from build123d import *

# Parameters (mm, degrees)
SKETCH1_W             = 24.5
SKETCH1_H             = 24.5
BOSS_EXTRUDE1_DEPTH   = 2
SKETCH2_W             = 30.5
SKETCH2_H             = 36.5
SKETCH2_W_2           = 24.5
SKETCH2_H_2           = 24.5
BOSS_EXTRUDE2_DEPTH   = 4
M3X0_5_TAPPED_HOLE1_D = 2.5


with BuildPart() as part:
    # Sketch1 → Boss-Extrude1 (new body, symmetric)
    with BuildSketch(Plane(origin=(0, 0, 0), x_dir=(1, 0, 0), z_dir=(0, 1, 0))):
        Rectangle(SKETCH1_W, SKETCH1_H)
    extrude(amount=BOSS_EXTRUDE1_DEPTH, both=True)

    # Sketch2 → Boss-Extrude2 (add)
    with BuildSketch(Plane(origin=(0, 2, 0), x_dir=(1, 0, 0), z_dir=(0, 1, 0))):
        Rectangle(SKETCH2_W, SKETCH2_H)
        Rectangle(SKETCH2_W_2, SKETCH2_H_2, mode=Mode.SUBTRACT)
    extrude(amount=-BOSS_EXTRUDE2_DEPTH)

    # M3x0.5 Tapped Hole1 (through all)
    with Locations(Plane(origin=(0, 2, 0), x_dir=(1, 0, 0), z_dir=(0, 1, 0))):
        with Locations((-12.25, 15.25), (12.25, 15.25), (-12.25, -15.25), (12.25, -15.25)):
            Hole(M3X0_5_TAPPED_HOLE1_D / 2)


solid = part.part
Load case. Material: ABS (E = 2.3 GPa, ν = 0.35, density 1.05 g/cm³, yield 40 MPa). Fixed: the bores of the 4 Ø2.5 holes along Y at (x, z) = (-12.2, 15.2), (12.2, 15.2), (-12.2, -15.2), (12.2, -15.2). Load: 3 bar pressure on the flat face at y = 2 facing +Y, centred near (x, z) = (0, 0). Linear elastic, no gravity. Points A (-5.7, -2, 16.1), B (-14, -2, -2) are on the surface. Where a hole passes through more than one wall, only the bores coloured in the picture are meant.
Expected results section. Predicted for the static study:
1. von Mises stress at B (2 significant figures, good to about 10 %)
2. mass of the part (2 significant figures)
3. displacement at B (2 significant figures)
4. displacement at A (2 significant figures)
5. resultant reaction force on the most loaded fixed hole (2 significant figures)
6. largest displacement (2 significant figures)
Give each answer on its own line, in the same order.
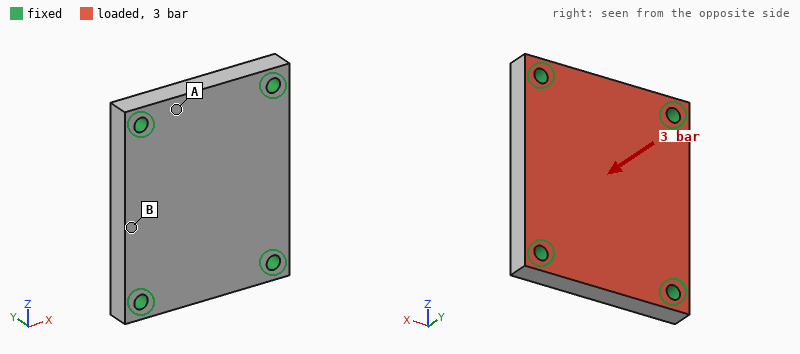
5.3 MPa
4.6 g
0.081 mm
0.027 mm
82 N
0.11 mm
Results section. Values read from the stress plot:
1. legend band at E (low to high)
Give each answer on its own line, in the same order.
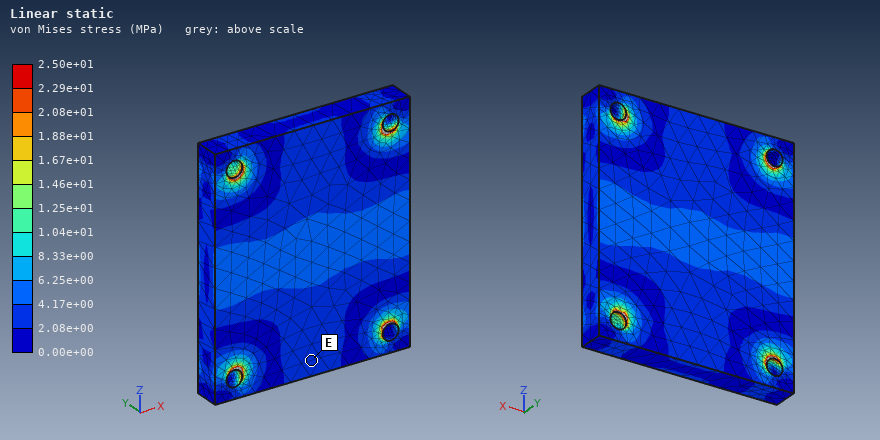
2.08e+00 to 4.17e+00 MPa
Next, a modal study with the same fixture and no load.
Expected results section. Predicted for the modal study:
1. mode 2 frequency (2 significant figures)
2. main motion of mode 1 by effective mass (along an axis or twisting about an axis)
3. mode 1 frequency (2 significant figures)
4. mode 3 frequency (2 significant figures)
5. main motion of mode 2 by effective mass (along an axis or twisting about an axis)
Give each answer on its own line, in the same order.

7000 Hz
along Y
4700 Hz
8900 Hz
twisting about Z
